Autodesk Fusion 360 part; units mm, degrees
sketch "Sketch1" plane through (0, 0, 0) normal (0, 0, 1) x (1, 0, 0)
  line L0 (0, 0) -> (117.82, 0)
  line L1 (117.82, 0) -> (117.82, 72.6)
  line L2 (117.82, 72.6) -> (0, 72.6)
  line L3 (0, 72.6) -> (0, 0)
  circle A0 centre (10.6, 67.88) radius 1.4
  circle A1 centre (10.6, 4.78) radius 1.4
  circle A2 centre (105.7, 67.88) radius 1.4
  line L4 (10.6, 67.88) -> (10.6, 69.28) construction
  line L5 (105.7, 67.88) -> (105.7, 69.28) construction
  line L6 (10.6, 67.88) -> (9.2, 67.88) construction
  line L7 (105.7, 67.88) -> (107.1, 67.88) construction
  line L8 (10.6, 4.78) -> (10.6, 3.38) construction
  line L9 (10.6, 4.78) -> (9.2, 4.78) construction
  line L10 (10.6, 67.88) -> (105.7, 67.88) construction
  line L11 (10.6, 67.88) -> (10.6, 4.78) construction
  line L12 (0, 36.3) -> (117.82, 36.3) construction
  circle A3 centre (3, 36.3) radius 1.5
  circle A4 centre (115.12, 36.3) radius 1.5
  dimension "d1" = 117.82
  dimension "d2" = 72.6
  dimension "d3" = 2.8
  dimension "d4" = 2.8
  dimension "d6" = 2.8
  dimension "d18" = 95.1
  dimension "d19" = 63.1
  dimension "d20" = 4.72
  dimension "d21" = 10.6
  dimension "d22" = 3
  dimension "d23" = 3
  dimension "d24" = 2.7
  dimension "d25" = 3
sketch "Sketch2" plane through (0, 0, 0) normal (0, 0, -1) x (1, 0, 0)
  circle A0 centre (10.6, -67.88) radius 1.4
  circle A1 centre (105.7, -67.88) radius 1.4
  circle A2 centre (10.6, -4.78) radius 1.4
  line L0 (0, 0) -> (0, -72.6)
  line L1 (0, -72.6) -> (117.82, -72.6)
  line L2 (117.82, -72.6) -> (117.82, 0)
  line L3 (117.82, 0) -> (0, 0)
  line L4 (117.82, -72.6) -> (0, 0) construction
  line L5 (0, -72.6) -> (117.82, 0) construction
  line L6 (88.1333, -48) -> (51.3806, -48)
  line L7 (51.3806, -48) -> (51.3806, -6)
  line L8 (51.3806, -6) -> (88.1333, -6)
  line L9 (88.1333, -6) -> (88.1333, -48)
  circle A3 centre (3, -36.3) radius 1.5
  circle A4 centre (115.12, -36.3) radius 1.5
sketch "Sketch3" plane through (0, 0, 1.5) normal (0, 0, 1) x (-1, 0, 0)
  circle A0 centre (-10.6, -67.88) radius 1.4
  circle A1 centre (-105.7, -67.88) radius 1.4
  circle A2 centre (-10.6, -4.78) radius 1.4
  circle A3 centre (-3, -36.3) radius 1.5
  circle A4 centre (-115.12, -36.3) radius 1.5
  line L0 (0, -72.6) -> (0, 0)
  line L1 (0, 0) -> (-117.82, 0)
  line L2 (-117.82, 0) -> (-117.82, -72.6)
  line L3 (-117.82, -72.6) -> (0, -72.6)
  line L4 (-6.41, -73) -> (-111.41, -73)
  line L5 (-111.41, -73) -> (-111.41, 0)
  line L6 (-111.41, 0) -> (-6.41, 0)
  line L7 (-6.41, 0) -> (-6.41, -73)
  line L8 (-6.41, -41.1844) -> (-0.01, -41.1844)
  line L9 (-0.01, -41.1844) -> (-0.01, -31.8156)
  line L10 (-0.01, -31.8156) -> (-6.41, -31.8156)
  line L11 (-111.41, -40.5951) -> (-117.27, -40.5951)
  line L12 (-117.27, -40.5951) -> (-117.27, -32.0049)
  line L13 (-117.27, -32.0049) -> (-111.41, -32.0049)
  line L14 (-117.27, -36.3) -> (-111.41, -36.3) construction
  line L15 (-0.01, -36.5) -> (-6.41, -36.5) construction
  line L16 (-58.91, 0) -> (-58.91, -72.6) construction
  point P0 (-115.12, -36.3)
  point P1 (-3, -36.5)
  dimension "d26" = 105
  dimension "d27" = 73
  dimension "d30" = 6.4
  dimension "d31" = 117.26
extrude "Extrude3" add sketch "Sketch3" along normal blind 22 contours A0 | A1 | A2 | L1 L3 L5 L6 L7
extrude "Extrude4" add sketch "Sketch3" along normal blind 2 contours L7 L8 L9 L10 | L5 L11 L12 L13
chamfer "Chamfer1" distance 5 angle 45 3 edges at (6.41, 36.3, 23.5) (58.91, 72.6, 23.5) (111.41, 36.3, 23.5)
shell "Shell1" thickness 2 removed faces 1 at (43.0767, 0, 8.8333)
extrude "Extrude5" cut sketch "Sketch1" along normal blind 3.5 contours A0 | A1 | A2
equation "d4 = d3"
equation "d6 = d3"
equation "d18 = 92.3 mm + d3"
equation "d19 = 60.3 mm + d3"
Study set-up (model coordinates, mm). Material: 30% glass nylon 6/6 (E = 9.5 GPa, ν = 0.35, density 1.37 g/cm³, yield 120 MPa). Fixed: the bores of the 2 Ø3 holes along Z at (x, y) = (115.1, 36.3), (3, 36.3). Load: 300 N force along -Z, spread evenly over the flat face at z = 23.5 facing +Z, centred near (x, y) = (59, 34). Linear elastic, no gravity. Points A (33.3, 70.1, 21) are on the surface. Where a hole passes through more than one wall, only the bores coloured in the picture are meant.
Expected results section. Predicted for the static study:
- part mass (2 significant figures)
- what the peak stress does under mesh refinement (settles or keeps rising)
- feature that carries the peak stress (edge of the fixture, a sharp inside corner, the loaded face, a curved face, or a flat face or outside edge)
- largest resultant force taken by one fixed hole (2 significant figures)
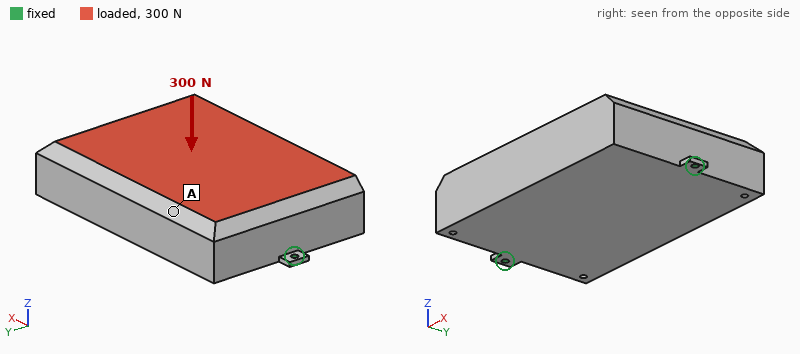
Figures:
230 g
keeps rising
edge of the fixture
180 N
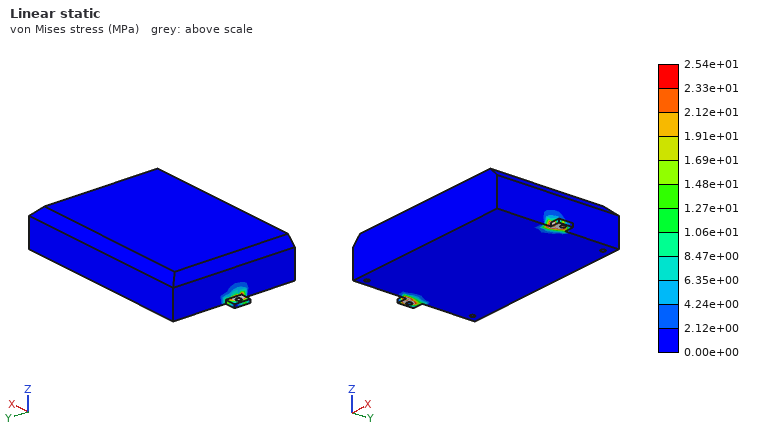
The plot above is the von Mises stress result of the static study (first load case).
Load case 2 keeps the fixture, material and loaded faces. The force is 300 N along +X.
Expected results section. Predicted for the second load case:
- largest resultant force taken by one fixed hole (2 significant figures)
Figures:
160 N
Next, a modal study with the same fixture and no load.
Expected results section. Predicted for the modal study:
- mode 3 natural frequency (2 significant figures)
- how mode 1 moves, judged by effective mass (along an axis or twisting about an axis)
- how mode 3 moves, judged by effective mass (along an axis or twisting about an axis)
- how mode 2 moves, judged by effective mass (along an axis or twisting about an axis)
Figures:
1600 Hz
along Y
along Y
along Z
